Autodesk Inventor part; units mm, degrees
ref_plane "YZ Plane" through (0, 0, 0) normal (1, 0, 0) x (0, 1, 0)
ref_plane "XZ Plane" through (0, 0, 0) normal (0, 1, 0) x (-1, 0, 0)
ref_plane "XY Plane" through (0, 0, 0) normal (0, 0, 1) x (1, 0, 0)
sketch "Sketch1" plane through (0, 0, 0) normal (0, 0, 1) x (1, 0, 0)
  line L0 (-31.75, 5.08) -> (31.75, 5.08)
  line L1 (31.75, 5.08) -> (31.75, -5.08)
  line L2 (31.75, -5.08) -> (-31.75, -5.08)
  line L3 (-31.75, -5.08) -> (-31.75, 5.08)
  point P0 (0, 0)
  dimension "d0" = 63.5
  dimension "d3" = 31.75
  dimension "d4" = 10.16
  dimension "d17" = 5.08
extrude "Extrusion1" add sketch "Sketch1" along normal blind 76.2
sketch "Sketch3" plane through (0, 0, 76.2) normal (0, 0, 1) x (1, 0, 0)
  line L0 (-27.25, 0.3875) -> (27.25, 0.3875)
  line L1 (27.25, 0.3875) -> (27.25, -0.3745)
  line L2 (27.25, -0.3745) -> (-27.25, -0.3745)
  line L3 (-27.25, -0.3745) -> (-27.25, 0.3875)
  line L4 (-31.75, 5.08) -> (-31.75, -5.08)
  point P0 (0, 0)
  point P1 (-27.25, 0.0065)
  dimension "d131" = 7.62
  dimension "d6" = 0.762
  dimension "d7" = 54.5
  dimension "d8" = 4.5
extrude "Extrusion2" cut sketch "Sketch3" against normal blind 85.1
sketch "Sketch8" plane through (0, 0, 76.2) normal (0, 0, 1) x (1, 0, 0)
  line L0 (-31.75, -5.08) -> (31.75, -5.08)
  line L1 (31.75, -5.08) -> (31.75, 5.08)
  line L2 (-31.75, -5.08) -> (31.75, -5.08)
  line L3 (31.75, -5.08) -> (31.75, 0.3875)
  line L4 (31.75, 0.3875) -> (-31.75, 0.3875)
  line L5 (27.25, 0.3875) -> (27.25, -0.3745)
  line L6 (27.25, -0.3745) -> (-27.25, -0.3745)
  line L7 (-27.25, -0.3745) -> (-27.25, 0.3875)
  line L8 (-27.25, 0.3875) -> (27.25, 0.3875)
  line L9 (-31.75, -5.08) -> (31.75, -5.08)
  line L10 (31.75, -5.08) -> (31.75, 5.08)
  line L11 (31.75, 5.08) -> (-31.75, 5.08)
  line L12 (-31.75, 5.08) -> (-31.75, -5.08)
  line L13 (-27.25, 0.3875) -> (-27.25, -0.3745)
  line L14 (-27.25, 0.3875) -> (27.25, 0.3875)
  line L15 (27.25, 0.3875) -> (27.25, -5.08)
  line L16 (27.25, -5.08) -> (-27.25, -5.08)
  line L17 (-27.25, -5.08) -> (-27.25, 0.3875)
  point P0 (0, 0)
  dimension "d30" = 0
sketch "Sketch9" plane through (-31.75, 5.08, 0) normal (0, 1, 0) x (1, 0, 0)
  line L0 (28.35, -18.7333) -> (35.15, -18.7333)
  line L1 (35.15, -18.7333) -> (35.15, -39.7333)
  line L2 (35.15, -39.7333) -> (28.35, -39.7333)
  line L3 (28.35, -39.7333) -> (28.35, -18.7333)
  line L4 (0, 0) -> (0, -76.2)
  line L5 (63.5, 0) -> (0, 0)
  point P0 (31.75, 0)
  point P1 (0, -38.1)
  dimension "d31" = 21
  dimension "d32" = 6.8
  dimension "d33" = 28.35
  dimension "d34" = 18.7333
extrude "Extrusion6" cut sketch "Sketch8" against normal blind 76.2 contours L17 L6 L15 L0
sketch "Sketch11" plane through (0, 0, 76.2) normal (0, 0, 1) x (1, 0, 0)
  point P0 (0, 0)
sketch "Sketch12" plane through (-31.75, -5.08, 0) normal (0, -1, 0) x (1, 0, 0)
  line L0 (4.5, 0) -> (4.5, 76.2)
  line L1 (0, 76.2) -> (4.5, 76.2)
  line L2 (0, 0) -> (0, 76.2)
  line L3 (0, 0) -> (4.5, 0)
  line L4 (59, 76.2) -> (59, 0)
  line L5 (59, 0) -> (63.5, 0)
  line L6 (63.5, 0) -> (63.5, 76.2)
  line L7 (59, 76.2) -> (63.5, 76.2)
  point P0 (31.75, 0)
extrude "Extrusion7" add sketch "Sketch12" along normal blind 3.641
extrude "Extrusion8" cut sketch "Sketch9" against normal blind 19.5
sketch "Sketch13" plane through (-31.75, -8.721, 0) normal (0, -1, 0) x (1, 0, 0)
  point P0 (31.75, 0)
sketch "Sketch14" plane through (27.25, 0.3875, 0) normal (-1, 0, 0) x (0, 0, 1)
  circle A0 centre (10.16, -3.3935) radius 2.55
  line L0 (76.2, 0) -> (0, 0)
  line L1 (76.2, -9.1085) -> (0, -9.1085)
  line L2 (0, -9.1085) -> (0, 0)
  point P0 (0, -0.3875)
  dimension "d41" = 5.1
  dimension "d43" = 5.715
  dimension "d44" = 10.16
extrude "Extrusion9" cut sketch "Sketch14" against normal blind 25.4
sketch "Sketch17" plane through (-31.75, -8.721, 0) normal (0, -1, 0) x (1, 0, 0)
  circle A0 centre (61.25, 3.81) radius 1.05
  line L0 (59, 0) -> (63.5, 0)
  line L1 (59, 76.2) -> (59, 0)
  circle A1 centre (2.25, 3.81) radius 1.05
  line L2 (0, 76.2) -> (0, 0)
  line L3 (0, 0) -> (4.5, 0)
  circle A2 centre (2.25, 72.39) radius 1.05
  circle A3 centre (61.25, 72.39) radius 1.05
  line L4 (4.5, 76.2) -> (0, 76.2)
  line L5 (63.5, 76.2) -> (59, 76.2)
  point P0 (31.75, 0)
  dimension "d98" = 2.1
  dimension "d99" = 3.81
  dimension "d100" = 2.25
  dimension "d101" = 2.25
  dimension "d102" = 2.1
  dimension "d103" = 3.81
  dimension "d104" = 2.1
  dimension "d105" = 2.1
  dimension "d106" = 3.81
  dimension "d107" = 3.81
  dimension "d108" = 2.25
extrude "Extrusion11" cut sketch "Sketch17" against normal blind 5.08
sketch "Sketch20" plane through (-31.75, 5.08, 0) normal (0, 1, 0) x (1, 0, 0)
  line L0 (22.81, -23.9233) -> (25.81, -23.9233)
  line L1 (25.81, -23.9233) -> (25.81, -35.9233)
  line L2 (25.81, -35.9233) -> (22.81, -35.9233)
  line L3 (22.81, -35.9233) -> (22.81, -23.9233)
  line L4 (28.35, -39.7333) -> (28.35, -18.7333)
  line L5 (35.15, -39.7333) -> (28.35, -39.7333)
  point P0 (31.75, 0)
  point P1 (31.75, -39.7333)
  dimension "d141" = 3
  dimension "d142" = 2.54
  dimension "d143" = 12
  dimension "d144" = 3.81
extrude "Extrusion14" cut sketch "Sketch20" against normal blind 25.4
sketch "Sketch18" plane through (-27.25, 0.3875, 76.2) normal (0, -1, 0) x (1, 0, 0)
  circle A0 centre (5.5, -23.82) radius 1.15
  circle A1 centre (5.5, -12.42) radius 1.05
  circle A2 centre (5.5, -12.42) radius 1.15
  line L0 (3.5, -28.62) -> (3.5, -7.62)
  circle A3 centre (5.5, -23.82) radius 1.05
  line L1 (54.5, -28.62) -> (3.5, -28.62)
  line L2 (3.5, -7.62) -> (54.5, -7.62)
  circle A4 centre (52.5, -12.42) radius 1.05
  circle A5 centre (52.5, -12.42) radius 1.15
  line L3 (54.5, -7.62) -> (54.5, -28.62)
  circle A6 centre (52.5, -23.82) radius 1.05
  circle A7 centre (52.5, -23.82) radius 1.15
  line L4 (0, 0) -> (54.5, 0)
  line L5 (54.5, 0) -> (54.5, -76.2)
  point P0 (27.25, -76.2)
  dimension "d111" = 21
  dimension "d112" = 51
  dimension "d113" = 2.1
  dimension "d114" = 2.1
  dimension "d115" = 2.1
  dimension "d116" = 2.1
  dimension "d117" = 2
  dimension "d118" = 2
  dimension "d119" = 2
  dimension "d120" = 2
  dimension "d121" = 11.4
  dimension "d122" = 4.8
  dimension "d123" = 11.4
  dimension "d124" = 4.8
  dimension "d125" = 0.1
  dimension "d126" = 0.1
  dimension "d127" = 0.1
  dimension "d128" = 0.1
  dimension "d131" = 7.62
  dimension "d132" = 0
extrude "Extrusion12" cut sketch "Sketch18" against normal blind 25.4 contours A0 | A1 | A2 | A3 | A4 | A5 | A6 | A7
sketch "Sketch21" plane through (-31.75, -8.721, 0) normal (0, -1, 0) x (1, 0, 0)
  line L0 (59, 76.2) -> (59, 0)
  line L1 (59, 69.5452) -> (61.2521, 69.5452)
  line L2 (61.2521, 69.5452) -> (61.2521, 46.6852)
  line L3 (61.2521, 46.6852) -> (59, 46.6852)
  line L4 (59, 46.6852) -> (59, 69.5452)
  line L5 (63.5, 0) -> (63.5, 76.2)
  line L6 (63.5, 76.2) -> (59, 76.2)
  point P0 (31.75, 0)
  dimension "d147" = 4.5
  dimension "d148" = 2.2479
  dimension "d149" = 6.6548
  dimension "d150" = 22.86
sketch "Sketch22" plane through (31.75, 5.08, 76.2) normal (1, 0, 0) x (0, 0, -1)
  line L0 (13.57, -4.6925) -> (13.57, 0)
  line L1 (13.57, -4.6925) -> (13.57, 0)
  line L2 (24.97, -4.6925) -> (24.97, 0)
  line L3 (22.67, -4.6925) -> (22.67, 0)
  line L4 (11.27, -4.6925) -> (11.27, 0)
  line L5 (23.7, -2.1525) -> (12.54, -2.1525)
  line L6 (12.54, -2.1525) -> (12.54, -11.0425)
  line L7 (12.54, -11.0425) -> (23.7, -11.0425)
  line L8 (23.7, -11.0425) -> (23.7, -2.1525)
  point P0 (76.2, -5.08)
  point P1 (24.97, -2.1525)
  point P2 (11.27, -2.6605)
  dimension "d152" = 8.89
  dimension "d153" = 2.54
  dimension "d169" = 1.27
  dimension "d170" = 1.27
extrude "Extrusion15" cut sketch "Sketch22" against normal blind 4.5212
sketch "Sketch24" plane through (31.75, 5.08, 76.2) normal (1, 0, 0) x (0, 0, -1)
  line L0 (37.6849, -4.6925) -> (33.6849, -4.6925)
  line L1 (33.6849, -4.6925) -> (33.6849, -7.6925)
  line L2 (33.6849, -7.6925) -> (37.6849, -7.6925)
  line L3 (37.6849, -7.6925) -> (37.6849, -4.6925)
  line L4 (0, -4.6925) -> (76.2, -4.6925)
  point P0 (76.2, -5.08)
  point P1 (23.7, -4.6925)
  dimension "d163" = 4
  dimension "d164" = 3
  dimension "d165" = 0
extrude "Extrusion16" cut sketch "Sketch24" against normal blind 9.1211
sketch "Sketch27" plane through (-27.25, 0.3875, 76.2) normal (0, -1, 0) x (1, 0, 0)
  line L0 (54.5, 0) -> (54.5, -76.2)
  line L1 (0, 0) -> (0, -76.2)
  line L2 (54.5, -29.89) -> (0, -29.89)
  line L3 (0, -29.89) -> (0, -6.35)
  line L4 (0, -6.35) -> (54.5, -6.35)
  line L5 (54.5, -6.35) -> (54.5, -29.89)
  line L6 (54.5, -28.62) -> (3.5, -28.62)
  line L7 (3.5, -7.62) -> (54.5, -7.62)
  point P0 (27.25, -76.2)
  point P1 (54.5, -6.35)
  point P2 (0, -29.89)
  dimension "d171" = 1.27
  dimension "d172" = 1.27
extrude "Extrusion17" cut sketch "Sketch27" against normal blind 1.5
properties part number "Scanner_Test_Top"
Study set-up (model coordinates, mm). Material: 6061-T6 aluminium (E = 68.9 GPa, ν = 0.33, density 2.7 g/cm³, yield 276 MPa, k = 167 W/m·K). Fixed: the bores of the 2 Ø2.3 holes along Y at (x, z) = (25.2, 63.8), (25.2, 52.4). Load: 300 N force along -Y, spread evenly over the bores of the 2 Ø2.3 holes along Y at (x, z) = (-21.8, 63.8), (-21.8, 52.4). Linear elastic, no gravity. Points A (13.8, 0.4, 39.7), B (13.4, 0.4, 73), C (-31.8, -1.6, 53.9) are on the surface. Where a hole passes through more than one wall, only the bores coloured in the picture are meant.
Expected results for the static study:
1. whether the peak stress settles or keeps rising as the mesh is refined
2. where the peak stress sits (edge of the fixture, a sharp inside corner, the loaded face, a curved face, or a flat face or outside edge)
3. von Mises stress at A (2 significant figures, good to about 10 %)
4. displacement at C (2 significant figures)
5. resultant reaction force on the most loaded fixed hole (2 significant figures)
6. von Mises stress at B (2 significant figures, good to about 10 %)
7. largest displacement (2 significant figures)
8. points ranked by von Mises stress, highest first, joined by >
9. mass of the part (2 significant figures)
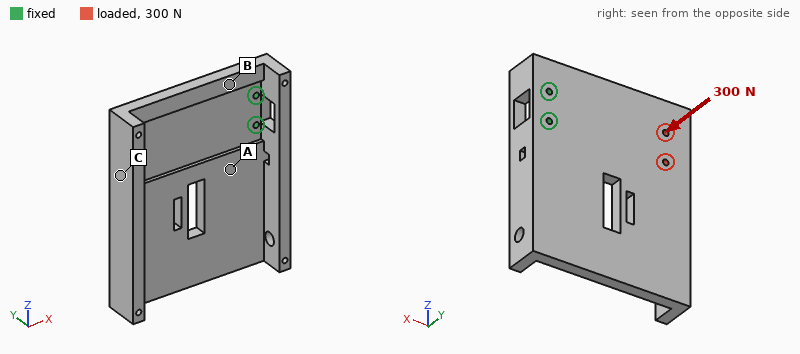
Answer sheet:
keeps rising
edge of the fixture
55 MPa
1.0 mm
210 N
110 MPa
1.1 mm
B > A > C
69 g
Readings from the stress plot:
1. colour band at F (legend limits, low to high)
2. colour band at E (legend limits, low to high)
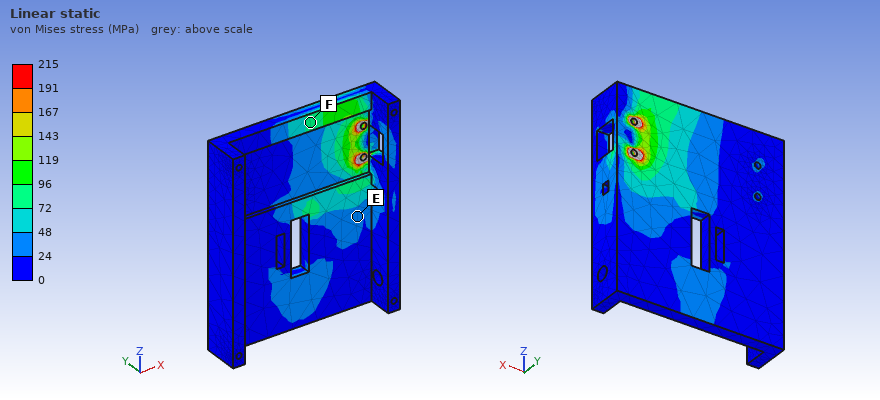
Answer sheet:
72 to 96 MPa
24 to 48 MPa
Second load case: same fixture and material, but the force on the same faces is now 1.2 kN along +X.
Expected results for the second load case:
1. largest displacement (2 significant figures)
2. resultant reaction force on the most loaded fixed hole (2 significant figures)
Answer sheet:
21 µm
600 N
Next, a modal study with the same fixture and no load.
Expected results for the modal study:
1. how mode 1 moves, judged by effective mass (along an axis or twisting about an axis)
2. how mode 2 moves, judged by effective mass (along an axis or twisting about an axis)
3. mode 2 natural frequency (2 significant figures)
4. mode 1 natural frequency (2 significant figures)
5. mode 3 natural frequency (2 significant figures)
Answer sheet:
along Y
twisting about X
1000 Hz
470 Hz
1700 Hz
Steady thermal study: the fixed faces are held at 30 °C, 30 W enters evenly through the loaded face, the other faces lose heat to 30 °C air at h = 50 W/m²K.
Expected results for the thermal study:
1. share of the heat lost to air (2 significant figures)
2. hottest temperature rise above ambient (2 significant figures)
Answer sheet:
43 %
45 K
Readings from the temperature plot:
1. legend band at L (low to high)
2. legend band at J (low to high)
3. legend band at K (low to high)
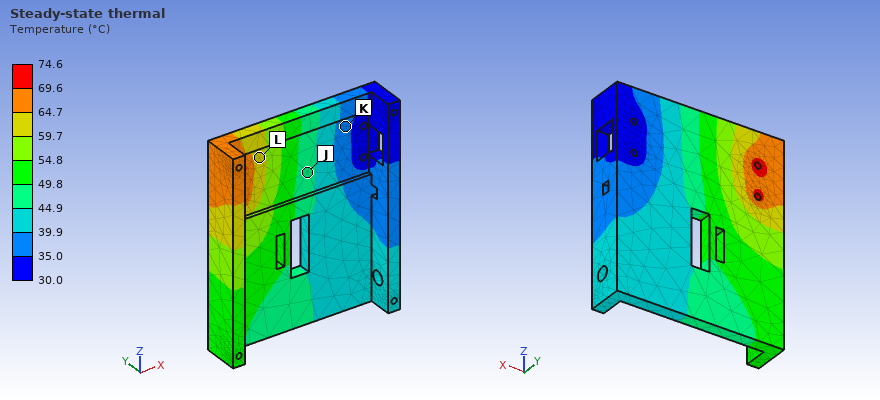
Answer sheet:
59.7 to 64.7 °C
44.9 to 49.8 °C
35.0 to 39.9 °C
